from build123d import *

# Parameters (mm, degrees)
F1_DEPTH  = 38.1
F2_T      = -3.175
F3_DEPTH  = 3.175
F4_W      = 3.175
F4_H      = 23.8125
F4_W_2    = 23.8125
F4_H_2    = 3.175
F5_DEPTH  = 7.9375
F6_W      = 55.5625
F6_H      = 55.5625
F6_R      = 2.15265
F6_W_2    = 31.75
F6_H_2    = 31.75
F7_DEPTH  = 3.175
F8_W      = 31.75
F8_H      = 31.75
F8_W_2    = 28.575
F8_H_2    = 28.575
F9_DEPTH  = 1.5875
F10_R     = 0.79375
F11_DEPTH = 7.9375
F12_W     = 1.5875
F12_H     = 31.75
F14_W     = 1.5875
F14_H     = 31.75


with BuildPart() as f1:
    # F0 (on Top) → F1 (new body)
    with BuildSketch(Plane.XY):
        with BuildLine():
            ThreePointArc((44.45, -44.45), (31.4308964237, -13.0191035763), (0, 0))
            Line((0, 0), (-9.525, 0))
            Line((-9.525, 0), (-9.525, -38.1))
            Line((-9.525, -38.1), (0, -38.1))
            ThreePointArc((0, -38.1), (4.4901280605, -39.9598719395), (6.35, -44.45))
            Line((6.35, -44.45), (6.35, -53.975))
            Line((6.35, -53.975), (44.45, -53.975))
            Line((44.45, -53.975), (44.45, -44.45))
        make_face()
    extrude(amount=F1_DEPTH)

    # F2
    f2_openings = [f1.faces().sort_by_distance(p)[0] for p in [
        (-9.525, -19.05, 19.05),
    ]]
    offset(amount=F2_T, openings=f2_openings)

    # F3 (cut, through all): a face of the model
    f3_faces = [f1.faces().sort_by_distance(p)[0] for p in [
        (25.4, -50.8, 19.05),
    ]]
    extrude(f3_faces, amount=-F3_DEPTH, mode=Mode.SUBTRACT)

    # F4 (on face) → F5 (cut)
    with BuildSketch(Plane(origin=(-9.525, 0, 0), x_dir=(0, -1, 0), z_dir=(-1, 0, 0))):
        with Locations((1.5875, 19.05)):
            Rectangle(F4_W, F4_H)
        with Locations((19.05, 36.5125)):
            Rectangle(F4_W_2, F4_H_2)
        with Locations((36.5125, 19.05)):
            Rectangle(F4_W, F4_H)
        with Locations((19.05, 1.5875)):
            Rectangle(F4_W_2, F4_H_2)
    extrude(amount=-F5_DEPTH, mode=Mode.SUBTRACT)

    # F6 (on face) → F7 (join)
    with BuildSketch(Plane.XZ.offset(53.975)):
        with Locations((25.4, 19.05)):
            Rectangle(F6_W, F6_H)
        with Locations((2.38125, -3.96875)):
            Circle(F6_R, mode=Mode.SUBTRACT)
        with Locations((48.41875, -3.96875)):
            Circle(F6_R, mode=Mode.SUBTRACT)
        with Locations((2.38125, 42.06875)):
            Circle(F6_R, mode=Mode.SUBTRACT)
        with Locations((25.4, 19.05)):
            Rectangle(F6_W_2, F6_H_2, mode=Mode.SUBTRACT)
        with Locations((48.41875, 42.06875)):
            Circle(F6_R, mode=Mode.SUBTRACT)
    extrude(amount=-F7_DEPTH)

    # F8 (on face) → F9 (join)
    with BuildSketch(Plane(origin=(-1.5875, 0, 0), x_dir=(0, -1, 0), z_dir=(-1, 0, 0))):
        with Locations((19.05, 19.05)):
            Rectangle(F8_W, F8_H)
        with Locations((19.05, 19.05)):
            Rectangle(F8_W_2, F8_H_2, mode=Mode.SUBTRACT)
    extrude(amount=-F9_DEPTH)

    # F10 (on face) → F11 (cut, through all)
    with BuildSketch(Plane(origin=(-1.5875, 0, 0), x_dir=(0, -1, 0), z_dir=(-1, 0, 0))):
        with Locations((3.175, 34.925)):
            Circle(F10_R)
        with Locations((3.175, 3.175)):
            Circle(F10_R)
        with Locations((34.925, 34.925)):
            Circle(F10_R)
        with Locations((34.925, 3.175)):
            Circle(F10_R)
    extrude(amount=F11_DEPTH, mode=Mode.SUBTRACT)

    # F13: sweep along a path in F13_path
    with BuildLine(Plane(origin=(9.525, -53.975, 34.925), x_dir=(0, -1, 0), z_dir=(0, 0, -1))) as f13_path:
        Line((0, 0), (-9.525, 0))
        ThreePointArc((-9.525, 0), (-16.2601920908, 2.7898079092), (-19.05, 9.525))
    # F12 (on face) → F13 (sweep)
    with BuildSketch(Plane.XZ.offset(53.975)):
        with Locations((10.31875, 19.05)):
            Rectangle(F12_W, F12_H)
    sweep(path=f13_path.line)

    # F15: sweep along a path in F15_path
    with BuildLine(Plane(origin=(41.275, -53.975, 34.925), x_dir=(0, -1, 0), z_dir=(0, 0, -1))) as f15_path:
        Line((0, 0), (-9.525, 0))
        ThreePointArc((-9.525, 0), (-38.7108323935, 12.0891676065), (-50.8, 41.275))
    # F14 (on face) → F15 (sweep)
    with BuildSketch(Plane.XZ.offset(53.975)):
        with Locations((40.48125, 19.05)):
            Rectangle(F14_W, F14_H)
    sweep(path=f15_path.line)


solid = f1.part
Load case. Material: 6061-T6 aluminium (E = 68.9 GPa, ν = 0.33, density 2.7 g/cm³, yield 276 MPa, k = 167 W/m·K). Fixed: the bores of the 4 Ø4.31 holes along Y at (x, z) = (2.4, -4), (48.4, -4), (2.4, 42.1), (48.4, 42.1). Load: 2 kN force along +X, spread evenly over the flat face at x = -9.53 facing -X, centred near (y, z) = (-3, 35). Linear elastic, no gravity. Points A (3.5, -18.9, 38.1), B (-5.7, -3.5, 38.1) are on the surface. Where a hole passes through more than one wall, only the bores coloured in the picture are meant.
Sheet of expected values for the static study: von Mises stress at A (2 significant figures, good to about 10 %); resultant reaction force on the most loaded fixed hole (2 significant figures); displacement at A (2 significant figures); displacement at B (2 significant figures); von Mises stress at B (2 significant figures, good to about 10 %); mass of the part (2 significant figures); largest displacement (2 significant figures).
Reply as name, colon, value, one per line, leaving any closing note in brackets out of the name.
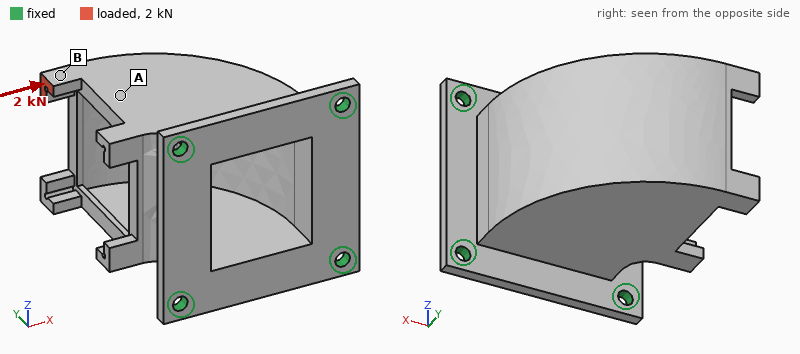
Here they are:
von Mises stress at A: 26 MPa
resultant reaction force on the most loaded fixed hole: 1.8 kN
displacement at A: 0.12 mm
displacement at B: 0.22 mm
von Mises stress at B: 61 MPa
mass of the part: 92 g
largest displacement: 0.25 mm
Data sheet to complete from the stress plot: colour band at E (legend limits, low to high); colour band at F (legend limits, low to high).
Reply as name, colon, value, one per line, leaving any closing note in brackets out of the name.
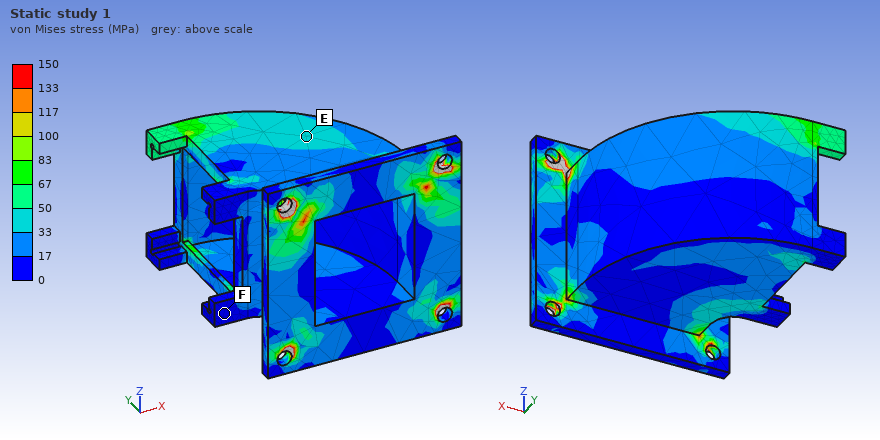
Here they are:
colour band at E: 33 to 50 MPa
colour band at F: 0 to 17 MPa
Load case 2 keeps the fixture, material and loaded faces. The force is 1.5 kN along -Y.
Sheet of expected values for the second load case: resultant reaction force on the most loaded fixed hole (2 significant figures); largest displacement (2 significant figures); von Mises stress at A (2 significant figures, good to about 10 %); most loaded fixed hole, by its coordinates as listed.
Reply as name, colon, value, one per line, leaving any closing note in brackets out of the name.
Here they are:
resultant reaction force on the most loaded fixed hole: 1.5 kN
largest displacement: 0.32 mm
von Mises stress at A: 41 MPa
most loaded fixed hole, by its coordinates as listed: (2.4, 42.1)
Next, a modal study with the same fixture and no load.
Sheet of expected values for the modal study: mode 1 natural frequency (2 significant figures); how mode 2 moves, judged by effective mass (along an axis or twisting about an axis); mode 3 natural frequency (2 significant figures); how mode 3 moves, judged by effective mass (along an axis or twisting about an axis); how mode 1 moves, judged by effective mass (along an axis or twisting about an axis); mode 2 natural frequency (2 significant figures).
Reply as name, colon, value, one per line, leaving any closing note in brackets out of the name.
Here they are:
mode 1 natural frequency: 2900 Hz
how mode 2 moves, judged by effective mass: along X
mode 3 natural frequency: 6300 Hz
how mode 3 moves, judged by effective mass: along Y
how mode 1 moves, judged by effective mass: along Z
mode 2 natural frequency: 3600 Hz
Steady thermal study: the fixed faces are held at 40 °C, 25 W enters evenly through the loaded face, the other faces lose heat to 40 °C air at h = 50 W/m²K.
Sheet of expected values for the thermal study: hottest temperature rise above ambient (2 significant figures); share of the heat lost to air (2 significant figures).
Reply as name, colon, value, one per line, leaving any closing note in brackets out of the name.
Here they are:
hottest temperature rise above ambient: 78 K
share of the heat lost to air: 38 %
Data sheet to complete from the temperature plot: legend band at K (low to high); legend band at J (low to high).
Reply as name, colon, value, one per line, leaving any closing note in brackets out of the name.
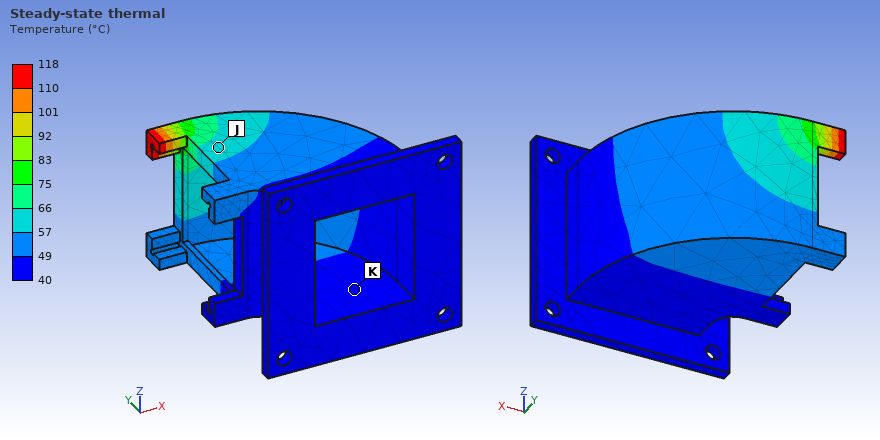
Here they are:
legend band at K: 40 to 49 °C
legend band at J: 57 to 66 °C
